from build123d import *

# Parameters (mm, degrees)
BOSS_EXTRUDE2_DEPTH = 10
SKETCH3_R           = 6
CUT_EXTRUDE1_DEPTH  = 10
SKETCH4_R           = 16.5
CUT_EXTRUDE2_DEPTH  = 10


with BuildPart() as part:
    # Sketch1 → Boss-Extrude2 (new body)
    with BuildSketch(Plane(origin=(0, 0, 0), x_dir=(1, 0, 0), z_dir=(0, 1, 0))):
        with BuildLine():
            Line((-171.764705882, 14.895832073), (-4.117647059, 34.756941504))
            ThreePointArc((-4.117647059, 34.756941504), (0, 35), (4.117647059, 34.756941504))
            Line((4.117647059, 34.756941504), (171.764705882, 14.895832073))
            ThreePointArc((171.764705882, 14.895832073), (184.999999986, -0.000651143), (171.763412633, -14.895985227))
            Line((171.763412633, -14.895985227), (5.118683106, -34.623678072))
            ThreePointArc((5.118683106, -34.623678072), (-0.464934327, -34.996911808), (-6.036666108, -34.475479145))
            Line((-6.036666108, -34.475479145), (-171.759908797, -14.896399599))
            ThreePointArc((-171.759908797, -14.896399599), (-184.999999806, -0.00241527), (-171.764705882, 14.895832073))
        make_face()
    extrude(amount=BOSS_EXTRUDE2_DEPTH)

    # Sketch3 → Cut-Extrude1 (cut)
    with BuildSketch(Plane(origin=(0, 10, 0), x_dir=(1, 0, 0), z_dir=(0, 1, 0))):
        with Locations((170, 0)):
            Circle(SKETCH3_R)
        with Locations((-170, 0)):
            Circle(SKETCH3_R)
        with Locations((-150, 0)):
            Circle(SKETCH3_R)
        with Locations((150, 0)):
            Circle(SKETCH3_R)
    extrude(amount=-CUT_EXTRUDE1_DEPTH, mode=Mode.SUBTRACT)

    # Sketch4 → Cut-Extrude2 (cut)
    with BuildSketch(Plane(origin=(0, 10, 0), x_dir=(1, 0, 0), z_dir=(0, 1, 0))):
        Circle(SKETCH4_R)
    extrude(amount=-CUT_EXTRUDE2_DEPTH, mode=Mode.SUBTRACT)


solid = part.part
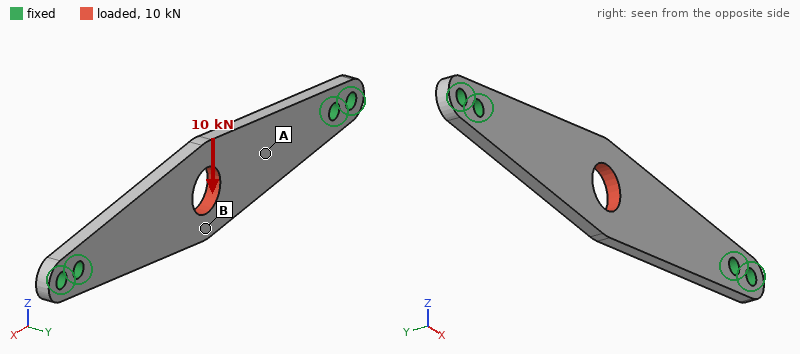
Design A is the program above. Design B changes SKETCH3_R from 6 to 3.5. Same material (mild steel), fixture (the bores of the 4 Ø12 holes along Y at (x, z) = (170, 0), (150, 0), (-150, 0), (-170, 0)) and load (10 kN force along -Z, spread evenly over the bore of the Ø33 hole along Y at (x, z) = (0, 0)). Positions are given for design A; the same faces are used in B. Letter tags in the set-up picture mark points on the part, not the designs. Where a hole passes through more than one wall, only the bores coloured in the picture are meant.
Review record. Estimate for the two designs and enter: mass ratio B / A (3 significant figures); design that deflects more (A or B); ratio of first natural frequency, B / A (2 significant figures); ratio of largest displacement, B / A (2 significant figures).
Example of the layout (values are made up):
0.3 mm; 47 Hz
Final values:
1.02; B; 0.95; 1.1
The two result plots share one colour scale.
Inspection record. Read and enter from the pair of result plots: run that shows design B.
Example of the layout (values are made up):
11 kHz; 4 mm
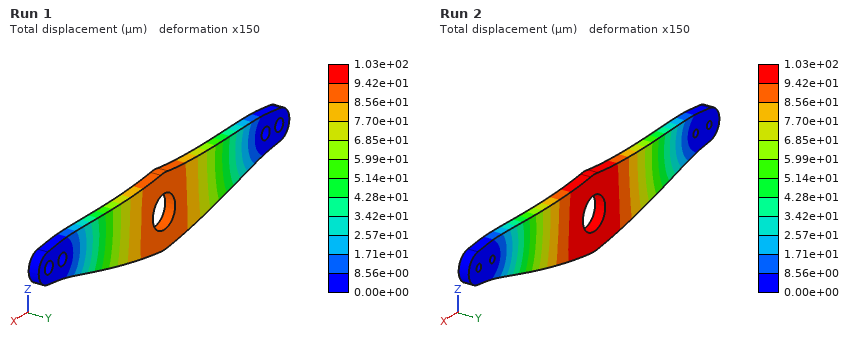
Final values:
Run 2
